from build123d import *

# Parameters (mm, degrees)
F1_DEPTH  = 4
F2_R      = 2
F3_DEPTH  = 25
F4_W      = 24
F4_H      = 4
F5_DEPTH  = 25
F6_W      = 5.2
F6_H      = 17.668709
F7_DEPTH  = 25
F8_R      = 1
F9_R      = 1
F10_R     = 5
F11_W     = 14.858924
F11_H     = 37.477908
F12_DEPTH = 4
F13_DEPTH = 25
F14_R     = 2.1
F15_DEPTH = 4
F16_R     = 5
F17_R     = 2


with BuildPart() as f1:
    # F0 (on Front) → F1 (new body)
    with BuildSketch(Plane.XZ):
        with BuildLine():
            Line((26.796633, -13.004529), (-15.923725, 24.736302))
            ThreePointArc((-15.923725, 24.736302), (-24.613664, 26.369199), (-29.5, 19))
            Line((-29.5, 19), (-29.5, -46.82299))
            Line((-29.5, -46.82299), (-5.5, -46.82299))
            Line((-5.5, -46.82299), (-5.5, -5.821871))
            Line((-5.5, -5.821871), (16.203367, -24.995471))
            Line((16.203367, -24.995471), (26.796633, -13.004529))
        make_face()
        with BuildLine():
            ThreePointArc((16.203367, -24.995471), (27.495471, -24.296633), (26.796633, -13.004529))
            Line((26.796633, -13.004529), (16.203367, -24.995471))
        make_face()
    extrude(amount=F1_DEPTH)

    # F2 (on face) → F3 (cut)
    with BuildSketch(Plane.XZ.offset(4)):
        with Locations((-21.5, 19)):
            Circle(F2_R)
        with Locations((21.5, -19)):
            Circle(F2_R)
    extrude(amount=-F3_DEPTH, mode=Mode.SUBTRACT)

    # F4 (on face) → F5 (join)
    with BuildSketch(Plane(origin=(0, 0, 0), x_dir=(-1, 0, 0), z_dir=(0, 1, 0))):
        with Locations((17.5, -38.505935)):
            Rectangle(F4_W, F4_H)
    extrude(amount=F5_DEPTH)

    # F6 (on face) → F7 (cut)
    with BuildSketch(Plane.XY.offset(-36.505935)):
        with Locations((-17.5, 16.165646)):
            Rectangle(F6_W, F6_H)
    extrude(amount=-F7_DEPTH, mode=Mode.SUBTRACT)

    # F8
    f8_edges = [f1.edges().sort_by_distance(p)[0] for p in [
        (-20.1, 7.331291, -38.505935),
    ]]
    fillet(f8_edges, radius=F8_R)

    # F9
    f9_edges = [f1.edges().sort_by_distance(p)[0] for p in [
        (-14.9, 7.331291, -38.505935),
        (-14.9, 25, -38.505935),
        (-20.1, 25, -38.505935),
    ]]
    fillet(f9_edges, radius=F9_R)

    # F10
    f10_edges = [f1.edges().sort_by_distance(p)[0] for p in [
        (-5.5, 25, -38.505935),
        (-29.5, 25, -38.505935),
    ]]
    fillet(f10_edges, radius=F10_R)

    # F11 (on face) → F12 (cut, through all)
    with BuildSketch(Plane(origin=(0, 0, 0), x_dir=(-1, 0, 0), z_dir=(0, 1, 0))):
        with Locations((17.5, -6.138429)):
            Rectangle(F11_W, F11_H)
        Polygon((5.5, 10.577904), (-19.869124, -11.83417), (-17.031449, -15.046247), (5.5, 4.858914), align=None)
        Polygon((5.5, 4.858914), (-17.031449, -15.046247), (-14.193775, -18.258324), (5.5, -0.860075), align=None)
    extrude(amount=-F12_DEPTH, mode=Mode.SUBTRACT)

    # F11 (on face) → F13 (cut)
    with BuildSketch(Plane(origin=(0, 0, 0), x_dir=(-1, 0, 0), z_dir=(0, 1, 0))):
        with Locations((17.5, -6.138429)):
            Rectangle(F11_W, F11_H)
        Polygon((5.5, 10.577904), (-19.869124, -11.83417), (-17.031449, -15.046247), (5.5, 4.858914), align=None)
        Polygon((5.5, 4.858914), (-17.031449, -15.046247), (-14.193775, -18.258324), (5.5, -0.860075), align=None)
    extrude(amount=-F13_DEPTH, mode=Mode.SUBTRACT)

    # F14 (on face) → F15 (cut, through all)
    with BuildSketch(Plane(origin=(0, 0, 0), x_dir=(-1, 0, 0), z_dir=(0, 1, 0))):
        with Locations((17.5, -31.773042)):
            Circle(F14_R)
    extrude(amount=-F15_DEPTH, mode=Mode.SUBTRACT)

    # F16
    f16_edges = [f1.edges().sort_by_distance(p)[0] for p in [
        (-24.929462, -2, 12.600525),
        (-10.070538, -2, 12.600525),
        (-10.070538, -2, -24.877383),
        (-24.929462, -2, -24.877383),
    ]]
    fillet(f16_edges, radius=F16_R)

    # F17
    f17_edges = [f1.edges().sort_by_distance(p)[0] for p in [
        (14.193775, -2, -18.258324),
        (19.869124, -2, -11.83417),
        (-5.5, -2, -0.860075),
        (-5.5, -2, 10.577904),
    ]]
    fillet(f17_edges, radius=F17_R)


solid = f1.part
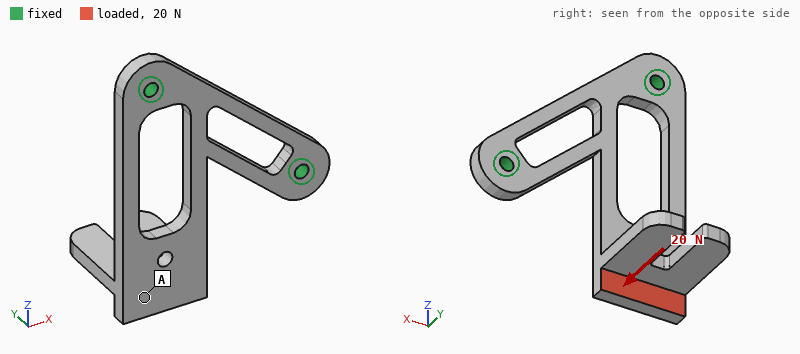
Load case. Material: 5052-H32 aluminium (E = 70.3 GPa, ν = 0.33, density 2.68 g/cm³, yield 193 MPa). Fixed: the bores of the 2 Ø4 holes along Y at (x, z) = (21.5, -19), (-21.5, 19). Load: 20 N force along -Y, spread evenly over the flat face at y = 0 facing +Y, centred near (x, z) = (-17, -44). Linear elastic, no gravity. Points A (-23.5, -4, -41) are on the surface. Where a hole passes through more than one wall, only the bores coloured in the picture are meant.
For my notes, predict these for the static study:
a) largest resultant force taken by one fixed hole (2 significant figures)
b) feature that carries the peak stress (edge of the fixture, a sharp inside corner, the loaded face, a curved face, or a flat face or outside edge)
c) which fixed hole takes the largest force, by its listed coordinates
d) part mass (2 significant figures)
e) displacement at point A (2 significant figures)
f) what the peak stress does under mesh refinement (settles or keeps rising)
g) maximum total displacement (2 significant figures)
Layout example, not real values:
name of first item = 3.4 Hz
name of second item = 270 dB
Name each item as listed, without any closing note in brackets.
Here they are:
largest resultant force taken by one fixed hole = 15 N
feature that carries the peak stress = a sharp inside corner
which fixed hole takes the largest force, by its listed coordinates = (21.5, -19)
part mass = 22 g
displacement at point A = 0.28 mm
what the peak stress does under mesh refinement = keeps rising
maximum total displacement = 0.35 mm
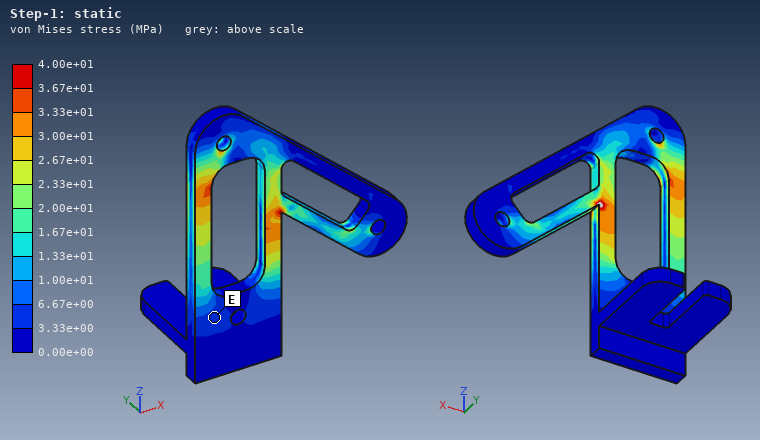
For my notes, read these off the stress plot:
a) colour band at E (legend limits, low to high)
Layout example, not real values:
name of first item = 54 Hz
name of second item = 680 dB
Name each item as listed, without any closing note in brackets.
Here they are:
colour band at E = 3.33e+00 to 6.67e+00 MPa
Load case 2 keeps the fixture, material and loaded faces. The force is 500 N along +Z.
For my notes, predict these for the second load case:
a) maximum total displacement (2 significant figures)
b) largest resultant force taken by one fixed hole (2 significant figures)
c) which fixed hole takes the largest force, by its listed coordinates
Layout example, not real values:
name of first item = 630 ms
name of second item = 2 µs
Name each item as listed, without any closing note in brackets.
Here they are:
maximum total displacement = 0.48 mm
largest resultant force taken by one fixed hole = 440 N
which fixed hole takes the largest force, by its listed coordinates = (-21.5, 19)
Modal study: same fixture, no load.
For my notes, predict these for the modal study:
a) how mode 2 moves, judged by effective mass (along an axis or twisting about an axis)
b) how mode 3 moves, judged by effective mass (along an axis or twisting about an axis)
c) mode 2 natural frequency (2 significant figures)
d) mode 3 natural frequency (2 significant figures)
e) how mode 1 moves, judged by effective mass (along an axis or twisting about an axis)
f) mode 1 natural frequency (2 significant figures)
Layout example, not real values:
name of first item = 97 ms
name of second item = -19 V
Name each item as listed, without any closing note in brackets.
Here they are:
how mode 2 moves, judged by effective mass = along X
how mode 3 moves, judged by effective mass = along X
mode 2 natural frequency = 1200 Hz
mode 3 natural frequency = 2000 Hz
how mode 1 moves, judged by effective mass = along Y
mode 1 natural frequency = 440 Hz
